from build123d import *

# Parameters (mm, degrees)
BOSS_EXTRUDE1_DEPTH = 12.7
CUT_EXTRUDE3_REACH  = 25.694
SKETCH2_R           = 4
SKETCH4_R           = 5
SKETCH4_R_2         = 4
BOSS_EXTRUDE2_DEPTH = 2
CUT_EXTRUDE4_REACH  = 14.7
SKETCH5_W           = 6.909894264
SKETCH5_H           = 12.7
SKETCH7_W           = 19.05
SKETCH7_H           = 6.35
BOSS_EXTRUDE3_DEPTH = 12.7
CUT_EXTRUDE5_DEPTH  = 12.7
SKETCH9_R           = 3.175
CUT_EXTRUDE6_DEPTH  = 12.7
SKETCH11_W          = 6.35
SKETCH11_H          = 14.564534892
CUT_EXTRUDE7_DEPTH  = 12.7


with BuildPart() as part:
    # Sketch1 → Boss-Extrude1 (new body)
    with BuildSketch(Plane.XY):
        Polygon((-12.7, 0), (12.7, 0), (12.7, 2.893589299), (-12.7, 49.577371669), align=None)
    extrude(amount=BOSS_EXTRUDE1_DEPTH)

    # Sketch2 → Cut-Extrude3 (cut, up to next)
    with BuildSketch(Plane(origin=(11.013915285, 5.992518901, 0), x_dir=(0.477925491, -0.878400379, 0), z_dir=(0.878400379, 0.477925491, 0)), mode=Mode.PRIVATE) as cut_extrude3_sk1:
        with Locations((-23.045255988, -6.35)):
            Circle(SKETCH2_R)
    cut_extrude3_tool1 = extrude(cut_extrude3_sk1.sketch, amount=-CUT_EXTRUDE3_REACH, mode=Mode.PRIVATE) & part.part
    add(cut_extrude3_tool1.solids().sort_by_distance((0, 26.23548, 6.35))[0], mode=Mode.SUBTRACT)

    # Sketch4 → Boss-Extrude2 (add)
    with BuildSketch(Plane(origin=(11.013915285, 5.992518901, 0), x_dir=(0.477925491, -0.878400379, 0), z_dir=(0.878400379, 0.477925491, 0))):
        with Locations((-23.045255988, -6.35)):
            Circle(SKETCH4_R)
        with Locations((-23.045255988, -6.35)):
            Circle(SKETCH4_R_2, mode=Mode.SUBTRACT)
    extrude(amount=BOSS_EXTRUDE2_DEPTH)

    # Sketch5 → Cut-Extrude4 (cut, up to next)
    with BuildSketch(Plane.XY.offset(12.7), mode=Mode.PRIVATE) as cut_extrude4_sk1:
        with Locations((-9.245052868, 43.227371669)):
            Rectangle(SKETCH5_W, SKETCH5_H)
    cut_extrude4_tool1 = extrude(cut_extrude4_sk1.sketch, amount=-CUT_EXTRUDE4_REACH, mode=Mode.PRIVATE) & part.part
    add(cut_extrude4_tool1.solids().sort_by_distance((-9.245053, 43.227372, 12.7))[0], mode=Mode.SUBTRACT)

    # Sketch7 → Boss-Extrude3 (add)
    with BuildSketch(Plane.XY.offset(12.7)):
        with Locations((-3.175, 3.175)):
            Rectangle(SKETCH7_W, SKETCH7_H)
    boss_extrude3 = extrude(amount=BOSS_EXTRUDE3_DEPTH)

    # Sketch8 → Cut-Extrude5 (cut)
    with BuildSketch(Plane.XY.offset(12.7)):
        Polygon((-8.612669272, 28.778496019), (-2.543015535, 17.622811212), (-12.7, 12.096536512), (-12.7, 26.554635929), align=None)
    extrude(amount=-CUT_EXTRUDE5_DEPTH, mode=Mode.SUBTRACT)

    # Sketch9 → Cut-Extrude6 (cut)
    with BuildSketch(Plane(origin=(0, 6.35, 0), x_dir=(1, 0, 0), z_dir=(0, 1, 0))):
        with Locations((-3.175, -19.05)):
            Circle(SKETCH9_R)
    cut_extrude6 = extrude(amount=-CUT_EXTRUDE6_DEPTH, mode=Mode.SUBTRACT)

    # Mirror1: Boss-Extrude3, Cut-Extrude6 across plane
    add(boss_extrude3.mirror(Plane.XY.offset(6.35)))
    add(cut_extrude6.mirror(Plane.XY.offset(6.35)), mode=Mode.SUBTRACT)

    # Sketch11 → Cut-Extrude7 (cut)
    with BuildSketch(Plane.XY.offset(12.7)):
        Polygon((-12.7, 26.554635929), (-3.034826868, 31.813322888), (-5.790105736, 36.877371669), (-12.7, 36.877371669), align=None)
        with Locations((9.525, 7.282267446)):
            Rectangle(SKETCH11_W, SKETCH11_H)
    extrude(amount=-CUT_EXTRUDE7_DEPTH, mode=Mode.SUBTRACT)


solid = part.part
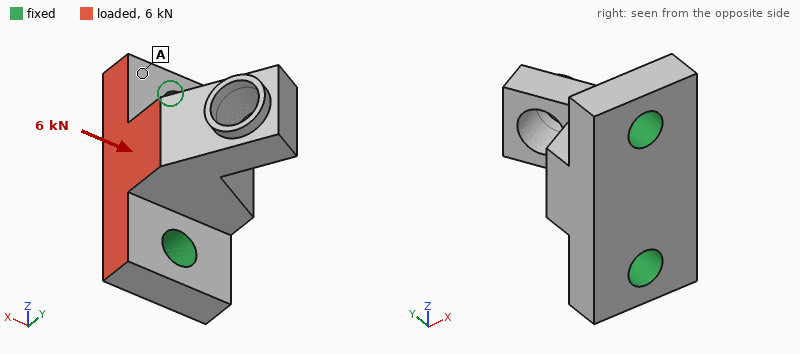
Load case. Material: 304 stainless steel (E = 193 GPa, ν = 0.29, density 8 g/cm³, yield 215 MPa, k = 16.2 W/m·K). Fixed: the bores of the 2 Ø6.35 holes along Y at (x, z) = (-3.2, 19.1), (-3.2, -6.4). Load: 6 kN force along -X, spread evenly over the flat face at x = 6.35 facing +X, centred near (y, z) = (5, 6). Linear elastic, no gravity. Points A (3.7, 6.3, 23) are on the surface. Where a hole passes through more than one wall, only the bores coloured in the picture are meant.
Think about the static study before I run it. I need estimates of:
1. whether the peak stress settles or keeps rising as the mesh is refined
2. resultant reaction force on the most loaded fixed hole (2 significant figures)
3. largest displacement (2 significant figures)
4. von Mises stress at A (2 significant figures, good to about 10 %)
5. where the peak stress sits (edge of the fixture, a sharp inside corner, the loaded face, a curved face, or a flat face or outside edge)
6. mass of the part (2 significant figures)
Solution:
keeps rising
3.0 kN
13 µm
18 MPa
edge of the fixture
60 g
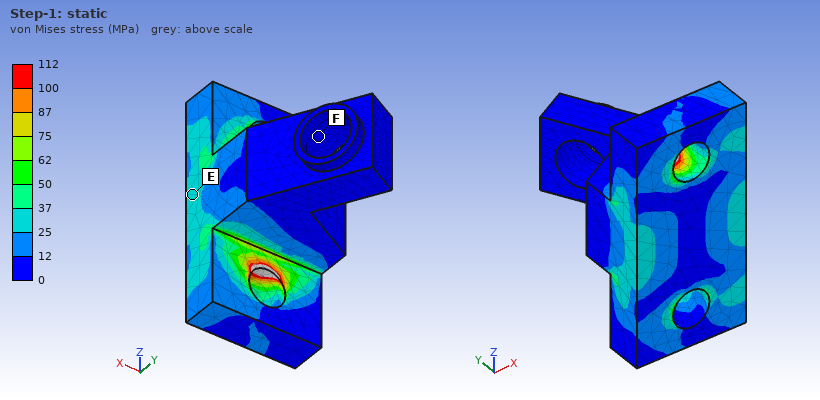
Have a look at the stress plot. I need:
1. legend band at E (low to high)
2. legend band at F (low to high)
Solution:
25 to 37 MPa
0 to 12 MPa
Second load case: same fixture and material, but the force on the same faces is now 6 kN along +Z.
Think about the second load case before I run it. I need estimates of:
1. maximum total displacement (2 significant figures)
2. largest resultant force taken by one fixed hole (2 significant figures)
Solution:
6.4 µm
3.5 kN
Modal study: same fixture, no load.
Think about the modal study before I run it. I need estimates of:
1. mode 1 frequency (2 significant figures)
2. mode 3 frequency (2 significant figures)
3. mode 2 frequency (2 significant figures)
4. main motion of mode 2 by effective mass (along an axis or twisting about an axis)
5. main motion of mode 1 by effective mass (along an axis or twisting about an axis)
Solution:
11 kHz
22 kHz
14 kHz
along Z
along X
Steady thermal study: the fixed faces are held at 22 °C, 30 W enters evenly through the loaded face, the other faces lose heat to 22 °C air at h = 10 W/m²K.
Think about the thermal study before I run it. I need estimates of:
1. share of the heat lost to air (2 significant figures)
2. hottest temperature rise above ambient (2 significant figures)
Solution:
3.3 %
77 K
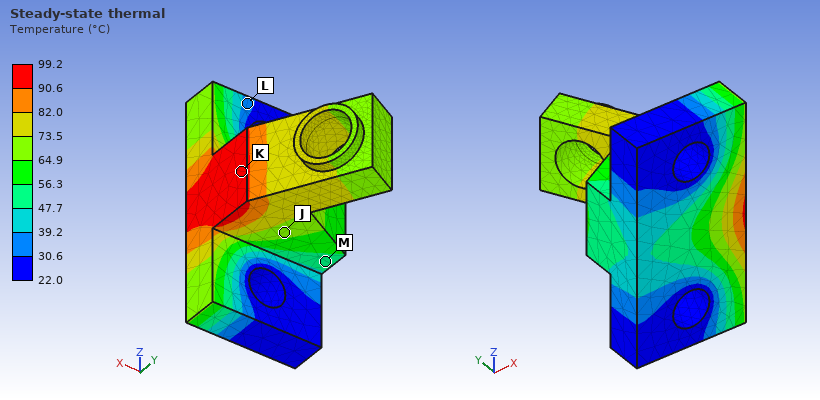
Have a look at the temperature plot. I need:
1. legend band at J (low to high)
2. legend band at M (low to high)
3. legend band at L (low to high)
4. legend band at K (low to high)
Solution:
64.9 to 73.5 °C
47.7 to 56.3 °C
30.6 to 39.2 °C
90.6 to 99.2 °C
